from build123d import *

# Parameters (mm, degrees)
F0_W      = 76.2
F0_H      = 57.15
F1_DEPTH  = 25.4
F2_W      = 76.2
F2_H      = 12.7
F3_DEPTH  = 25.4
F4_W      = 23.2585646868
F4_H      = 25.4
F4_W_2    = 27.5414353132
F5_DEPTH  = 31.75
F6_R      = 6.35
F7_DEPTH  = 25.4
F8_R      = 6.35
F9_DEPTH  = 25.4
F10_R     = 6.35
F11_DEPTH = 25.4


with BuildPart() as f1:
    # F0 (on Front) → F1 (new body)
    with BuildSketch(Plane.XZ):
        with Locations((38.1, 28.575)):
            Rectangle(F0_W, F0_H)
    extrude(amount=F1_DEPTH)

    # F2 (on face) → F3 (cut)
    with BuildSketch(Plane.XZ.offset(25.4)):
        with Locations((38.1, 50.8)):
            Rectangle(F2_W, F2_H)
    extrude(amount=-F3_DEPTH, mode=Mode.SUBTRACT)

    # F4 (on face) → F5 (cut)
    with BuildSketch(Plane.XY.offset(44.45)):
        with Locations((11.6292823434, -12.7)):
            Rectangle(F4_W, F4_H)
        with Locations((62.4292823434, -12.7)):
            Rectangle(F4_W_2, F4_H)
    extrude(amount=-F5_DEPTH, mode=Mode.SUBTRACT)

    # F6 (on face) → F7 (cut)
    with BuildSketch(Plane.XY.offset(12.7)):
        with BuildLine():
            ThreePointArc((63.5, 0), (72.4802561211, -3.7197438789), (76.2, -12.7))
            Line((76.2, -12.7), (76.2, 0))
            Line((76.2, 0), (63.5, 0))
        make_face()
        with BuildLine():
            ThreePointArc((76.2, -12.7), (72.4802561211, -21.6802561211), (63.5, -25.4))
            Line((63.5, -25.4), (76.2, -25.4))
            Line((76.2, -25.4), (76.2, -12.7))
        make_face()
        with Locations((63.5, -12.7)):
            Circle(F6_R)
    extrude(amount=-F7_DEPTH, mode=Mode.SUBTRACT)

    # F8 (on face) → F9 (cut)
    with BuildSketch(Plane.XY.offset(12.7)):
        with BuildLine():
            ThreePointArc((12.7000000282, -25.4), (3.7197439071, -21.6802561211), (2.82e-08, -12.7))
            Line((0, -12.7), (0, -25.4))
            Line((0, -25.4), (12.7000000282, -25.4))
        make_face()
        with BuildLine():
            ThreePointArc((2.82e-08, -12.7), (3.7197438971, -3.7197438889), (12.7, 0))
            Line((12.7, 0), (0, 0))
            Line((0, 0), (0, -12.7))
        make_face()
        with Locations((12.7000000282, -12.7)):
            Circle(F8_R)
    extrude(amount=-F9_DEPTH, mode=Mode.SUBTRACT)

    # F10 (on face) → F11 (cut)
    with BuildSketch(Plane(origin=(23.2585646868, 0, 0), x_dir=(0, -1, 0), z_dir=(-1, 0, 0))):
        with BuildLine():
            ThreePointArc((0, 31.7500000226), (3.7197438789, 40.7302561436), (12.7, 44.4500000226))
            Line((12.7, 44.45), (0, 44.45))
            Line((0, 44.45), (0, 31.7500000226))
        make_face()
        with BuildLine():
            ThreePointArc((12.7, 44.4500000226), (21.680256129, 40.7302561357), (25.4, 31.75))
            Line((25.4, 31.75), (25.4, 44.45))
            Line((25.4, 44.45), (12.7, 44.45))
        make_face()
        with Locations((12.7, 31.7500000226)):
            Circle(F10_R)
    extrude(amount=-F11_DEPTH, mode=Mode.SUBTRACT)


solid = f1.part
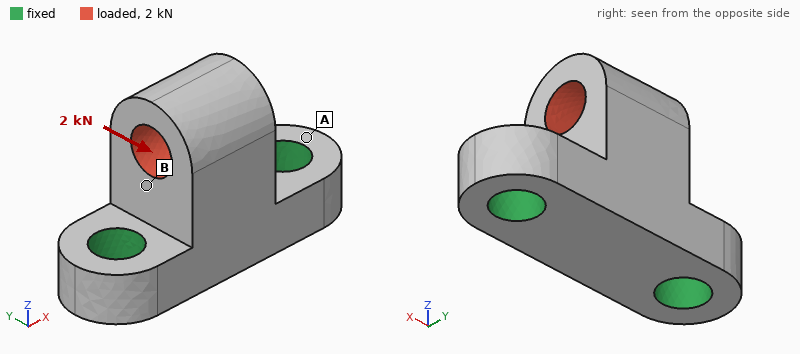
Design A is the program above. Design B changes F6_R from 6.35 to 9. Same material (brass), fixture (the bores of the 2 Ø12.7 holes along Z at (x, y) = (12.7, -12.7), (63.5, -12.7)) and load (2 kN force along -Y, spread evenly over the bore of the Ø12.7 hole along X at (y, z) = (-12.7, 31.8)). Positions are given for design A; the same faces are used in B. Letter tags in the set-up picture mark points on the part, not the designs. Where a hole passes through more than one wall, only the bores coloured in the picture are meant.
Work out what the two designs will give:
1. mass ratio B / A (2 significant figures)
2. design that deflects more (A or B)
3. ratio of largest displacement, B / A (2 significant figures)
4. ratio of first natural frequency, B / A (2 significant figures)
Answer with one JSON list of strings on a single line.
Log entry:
["0.95", "A", "0.90", "1.1"]
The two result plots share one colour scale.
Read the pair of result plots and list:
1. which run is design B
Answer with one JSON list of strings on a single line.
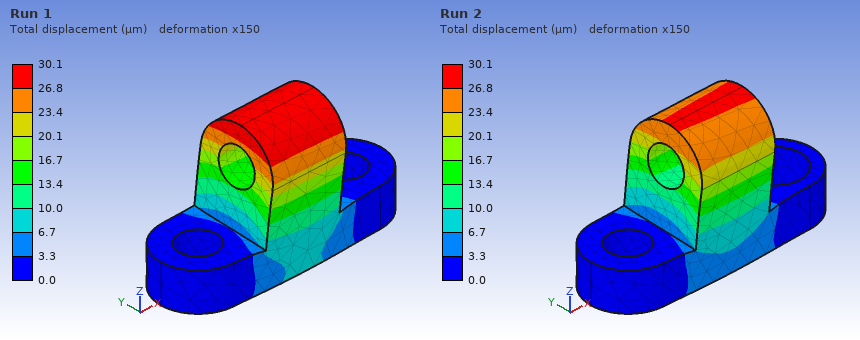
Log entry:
["Run 2"]
